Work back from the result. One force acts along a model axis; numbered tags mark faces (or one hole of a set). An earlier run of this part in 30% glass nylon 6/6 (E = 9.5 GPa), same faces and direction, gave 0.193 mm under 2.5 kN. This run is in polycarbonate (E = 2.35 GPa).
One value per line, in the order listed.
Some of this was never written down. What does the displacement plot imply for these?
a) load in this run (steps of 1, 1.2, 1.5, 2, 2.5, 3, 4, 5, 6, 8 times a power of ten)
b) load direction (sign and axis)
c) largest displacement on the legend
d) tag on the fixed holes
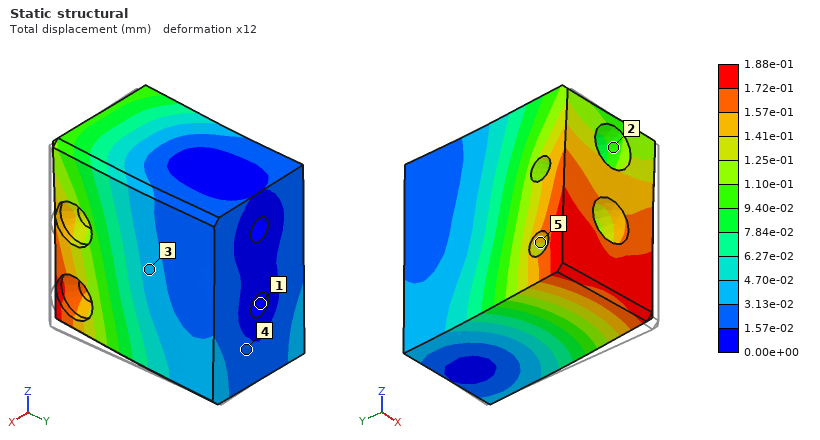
600 N
-X
1.88e-01 mm
1
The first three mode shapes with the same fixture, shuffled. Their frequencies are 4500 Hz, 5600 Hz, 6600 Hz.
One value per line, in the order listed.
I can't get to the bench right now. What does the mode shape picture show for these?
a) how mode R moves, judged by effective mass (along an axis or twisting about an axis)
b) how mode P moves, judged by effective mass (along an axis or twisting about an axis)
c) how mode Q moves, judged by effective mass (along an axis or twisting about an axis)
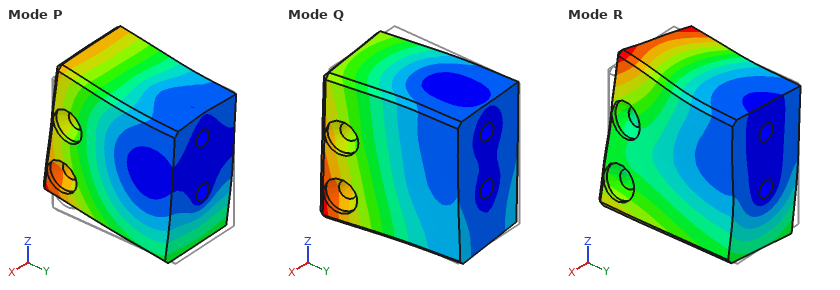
twisting about Y
along Z
along X
